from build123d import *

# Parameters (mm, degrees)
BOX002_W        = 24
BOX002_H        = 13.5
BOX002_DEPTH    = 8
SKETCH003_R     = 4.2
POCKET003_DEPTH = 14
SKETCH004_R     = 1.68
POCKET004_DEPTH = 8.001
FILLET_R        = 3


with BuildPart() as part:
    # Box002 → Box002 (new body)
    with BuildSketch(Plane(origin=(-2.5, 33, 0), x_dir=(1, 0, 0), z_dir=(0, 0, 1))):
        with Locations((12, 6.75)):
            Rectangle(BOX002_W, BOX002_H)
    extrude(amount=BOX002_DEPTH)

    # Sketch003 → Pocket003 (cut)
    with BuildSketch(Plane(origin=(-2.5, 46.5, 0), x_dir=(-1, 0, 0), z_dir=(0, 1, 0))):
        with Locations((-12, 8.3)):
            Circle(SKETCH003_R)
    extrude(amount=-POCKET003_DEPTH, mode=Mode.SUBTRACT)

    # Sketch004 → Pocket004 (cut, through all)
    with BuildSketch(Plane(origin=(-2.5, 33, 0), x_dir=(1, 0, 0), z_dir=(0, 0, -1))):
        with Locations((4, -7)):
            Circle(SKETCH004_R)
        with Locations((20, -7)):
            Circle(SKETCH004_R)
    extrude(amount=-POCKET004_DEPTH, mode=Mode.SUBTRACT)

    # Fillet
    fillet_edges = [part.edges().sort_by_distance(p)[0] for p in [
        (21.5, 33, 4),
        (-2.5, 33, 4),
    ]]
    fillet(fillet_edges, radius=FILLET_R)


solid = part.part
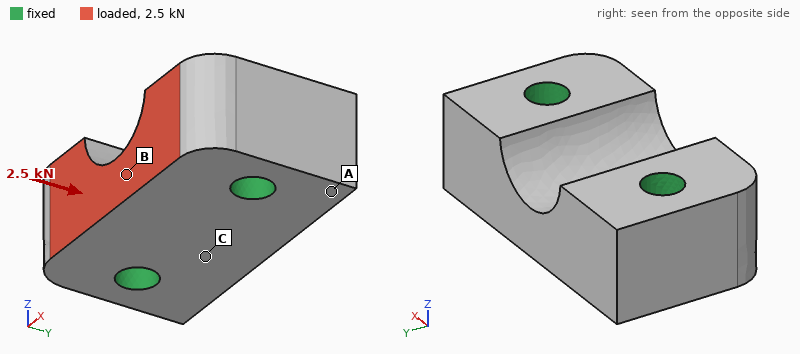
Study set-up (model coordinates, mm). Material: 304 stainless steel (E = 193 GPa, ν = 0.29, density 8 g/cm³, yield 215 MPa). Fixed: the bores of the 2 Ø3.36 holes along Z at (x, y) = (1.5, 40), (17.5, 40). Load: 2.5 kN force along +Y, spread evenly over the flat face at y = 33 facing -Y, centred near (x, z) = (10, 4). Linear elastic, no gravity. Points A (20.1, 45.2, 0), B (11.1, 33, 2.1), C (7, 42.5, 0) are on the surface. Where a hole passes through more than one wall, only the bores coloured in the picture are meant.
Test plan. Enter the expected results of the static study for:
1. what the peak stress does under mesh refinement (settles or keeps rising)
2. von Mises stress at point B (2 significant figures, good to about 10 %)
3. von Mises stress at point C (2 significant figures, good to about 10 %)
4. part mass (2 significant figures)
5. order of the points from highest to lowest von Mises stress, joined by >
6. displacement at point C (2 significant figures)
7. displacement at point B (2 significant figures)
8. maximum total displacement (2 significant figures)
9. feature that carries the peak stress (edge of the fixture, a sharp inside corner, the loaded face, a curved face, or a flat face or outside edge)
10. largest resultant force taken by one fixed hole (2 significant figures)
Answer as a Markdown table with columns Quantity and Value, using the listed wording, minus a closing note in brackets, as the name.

| Quantity | Value |
|---|---|
| what the peak stress does under mesh refinement | keeps rising |
| von Mises stress at point B | 21 MPa |
| von Mises stress at point C | 13 MPa |
| part mass | 17 g |
| order of the points from highest to lowest von Mises stress, joined by > | B > C > A |
| displacement at point C | 0.71 µm |
| displacement at point B | 1.3 µm |
| maximum total displacement | 1.6 µm |
| feature that carries the peak stress | edge of the fixture |
| largest resultant force taken by one fixed hole | 1.3 kN |
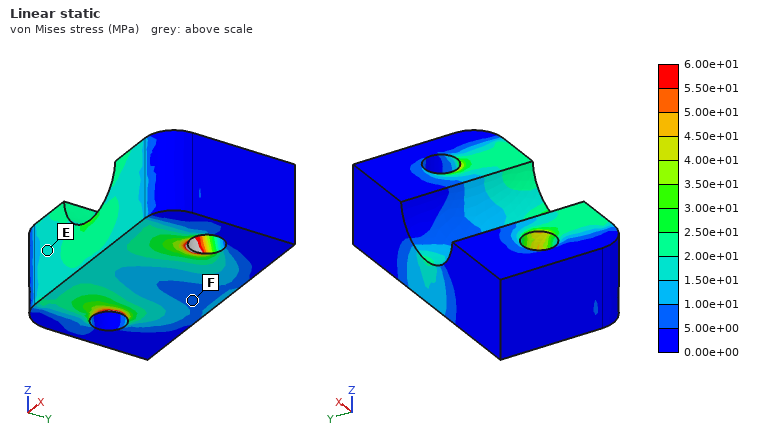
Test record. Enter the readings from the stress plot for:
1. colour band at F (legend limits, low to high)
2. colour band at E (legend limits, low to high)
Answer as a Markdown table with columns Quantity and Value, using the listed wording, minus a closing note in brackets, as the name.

| Quantity | Value |
|---|---|
| colour band at F | 5.00e+00 to 1.00e+01 MPa |
| colour band at E | 1.50e+01 to 2.00e+01 MPa |
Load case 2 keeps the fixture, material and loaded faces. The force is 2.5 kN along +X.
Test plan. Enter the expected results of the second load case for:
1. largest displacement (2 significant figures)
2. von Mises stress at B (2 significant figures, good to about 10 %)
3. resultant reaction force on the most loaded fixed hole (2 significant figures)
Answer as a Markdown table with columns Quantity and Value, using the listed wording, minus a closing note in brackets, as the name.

| Quantity | Value |
|---|---|
| largest displacement | 2.9 µm |
| von Mises stress at B | 40 MPa |
| resultant reaction force on the most loaded fixed hole | 1.5 kN |
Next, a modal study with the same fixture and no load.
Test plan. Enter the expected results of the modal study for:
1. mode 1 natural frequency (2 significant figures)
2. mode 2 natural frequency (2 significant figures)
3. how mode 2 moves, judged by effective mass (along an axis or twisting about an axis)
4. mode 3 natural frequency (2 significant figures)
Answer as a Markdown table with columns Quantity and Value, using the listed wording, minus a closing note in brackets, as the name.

| Quantity | Value |
|---|---|
| mode 1 natural frequency | 70 kHz |
| mode 2 natural frequency | 77 kHz |
| how mode 2 moves, judged by effective mass | along Z |
| mode 3 natural frequency | 84 kHz |
